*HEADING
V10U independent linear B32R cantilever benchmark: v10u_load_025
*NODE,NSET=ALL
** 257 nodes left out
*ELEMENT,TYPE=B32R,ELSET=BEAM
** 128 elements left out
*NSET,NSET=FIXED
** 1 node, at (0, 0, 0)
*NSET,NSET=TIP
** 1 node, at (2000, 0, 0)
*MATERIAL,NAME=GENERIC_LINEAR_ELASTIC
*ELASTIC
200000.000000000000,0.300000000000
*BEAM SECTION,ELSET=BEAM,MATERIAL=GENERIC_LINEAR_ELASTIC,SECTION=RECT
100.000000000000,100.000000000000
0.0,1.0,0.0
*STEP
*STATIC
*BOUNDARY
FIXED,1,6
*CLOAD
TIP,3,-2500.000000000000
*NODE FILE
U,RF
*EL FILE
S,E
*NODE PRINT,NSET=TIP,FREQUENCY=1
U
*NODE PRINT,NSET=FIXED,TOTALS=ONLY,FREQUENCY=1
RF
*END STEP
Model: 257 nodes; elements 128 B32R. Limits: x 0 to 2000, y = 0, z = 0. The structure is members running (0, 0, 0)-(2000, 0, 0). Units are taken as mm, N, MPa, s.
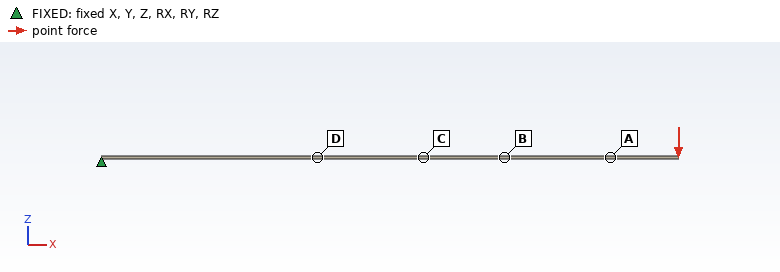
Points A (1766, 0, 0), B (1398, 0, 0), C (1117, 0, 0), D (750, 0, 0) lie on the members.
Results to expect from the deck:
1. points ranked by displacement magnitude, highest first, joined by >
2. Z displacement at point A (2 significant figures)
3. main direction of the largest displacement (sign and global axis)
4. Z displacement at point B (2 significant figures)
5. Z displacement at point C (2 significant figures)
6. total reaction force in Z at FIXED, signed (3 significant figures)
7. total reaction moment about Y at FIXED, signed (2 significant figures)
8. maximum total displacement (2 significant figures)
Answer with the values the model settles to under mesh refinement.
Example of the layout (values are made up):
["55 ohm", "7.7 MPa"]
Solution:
["A > B > C > D", "-3.3 mm", "-Z", "-2.3 mm", "-1.5 mm", "2500 N", "-5.0e+06 N·mm", "4.0 mm"]
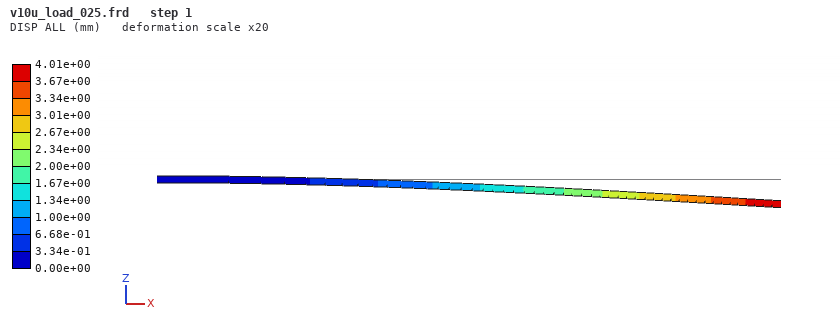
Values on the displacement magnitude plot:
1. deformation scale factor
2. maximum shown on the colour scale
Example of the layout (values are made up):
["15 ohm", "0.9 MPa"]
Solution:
["20", "4.01e+00 mm"]
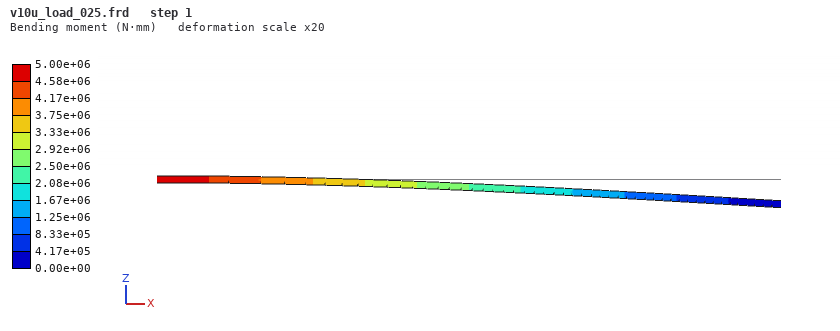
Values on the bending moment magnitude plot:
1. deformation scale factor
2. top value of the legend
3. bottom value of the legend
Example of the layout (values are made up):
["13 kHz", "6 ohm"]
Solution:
["20", "5.00e+06 N·mm", "0.00e+00 N·mm"]
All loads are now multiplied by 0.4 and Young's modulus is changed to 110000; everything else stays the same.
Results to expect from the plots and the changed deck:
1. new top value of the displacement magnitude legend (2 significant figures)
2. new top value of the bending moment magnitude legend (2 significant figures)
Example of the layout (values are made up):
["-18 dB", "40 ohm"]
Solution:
["2.9 mm", "2.0e+06 N·mm"]
